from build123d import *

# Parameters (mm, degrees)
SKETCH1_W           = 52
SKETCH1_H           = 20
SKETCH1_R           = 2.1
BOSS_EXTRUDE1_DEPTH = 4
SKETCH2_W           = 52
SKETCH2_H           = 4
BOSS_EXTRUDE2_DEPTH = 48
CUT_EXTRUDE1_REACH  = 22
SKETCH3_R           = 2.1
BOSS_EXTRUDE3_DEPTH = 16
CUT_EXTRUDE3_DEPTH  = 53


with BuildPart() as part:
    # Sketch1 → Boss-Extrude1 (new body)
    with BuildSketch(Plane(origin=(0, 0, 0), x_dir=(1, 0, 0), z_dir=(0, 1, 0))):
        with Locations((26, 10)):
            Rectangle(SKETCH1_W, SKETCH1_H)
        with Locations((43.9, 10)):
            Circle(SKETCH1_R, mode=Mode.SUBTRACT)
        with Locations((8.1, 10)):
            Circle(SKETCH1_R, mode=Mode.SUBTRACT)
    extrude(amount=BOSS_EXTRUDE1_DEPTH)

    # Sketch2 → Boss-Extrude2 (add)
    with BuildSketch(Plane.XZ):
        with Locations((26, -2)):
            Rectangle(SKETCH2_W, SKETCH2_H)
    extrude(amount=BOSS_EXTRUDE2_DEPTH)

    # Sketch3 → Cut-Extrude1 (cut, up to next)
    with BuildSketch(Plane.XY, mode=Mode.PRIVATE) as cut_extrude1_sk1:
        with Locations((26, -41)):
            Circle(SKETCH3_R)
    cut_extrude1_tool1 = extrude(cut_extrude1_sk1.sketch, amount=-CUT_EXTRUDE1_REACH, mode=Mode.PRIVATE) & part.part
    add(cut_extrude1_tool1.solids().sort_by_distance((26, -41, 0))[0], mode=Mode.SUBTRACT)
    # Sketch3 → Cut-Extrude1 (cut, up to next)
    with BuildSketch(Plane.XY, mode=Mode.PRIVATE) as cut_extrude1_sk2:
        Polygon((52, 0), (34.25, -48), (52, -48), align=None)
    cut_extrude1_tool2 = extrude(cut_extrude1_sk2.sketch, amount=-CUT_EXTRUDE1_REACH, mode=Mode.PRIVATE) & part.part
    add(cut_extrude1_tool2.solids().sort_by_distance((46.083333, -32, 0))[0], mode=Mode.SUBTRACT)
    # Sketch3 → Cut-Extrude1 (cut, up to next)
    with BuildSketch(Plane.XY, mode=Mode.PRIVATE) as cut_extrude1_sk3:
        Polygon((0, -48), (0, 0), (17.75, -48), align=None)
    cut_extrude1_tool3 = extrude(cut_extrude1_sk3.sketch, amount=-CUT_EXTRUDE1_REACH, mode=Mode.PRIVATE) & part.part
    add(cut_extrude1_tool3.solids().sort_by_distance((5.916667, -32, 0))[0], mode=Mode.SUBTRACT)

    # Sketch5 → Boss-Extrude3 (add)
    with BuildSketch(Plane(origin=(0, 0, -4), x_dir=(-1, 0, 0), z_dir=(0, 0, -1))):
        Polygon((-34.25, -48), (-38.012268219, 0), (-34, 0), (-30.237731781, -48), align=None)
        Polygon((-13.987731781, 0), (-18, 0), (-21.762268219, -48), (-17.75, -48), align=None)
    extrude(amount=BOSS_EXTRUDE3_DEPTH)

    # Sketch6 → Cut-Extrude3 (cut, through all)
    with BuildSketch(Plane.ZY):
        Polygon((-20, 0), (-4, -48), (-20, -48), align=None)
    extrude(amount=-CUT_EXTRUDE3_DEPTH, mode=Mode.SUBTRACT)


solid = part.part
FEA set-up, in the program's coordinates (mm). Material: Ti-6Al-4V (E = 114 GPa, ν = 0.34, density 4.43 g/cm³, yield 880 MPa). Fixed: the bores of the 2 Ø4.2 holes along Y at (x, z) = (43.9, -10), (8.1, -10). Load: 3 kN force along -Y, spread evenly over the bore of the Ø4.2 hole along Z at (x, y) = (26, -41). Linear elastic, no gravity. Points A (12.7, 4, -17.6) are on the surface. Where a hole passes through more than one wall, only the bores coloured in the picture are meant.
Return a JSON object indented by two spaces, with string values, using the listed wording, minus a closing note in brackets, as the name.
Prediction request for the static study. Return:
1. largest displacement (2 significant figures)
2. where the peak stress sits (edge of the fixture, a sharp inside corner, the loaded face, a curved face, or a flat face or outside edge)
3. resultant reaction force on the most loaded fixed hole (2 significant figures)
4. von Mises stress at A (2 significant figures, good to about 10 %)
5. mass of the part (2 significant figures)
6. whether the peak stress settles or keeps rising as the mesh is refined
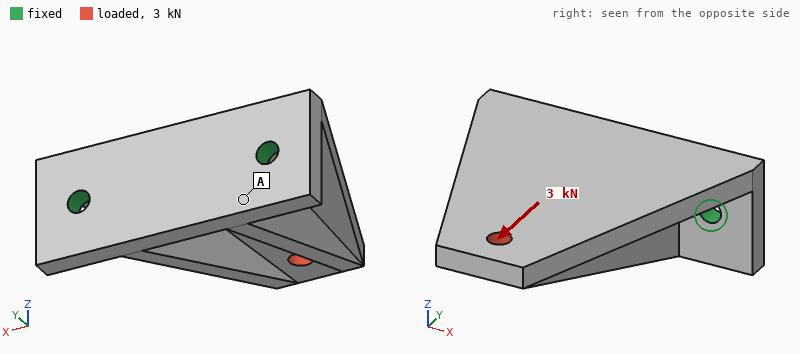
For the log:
{
  "largest displacement": "0.14 mm",
  "where the peak stress sits": "edge of the fixture",
  "resultant reaction force on the most loaded fixed hole": "1.5 kN",
  "von Mises stress at A": "29 MPa",
  "mass of the part": "60 g",
  "whether the peak stress settles or keeps rising as the mesh is refined": "keeps rising"
}
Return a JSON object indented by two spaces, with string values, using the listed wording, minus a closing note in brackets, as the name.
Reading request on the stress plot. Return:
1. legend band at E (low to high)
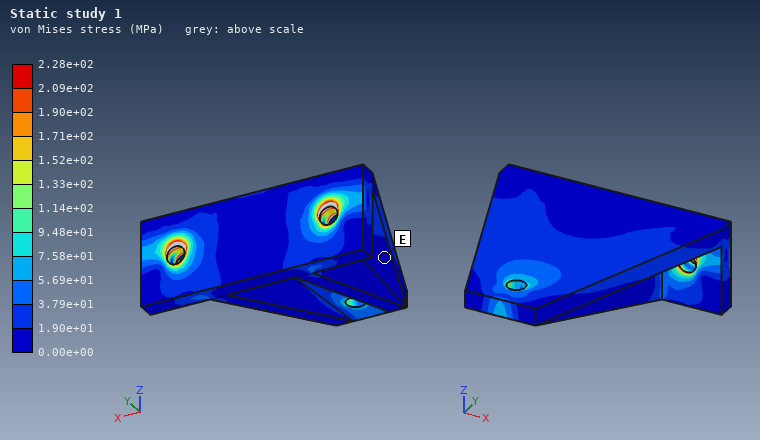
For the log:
{
  "legend band at E": "0.00e+00 to 1.90e+01 MPa"
}
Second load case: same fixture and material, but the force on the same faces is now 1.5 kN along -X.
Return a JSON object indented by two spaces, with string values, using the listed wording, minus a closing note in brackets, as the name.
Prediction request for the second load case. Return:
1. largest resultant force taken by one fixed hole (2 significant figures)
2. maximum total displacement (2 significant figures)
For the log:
{
  "largest resultant force taken by one fixed hole": "2.0 kN",
  "maximum total displacement": "64 µm"
}
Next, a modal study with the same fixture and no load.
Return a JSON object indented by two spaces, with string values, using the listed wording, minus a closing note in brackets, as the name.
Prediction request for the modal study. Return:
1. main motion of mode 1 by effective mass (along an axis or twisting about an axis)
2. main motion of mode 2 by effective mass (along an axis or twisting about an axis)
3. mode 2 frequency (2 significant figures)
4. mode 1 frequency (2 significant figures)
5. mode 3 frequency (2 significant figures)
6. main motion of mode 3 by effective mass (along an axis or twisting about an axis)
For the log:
{
  "main motion of mode 1 by effective mass": "along Z",
  "main motion of mode 2 by effective mass": "along X",
  "mode 2 frequency": "6100 Hz",
  "mode 1 frequency": "2600 Hz",
  "mode 3 frequency": "9600 Hz",
  "main motion of mode 3 by effective mass": "along X"
}
